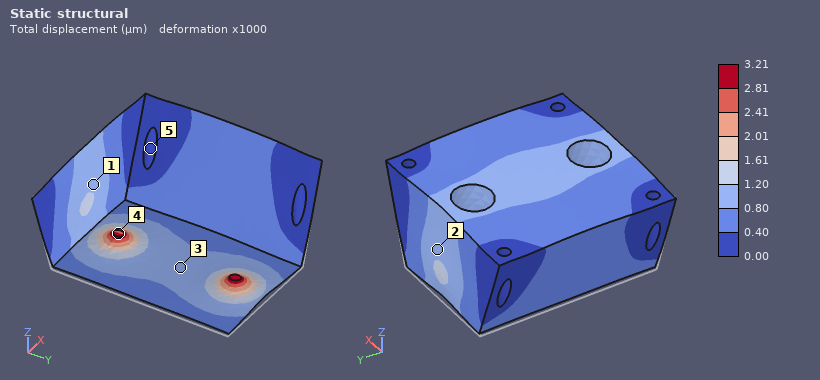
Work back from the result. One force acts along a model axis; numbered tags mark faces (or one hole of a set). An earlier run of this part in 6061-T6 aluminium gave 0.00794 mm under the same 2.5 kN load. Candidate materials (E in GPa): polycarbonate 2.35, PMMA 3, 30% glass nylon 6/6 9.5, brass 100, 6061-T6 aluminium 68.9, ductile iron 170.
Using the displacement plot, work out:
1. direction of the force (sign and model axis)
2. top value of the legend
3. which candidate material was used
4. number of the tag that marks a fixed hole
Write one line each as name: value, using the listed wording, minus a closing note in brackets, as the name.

direction of the force: +Z
top value of the legend: 3.21 µm
which candidate material was used: ductile iron
number of the tag that marks a fixed hole: 5
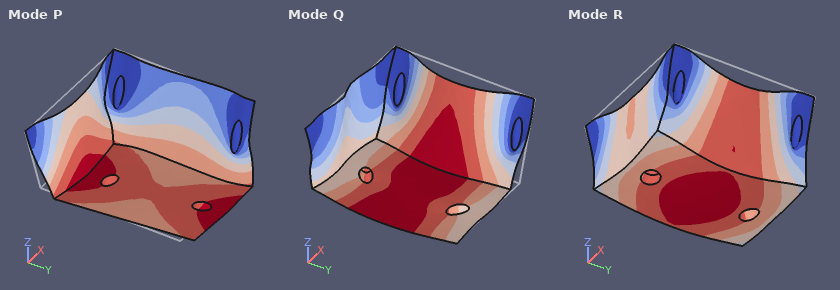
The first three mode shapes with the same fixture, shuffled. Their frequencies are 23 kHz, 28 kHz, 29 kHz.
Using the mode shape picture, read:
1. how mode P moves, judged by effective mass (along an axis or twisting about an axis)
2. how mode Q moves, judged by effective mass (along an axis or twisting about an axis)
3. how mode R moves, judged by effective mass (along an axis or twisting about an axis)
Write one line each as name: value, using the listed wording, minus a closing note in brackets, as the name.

how mode P moves, judged by effective mass: along Y
how mode Q moves, judged by effective mass: along X
how mode R moves, judged by effective mass: along Z
